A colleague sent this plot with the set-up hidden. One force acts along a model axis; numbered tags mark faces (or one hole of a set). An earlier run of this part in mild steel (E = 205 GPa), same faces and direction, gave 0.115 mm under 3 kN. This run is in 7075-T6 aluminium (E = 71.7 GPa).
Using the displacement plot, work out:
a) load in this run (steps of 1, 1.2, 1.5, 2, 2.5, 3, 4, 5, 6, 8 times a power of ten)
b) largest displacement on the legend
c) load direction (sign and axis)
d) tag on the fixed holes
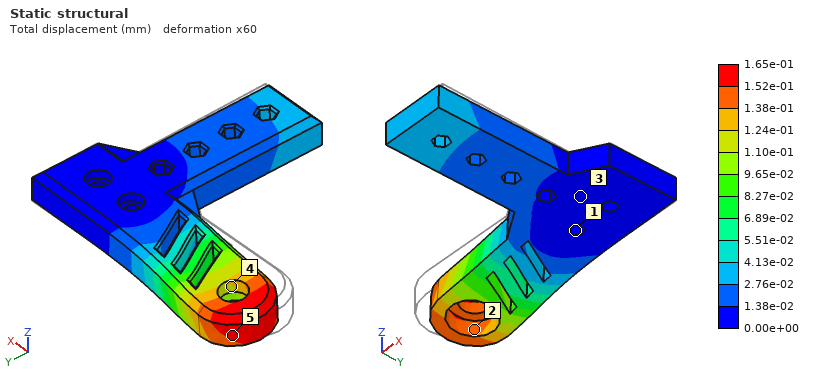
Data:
1.5 kN
1.65e-01 mm
+Y
1
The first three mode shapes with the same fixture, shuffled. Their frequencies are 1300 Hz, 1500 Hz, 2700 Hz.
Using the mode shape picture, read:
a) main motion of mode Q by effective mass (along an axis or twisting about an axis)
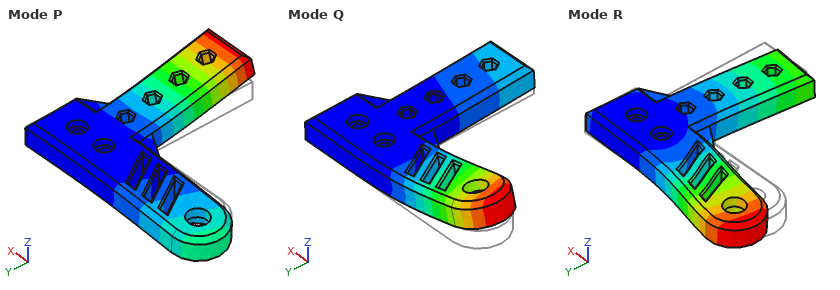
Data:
along Z
